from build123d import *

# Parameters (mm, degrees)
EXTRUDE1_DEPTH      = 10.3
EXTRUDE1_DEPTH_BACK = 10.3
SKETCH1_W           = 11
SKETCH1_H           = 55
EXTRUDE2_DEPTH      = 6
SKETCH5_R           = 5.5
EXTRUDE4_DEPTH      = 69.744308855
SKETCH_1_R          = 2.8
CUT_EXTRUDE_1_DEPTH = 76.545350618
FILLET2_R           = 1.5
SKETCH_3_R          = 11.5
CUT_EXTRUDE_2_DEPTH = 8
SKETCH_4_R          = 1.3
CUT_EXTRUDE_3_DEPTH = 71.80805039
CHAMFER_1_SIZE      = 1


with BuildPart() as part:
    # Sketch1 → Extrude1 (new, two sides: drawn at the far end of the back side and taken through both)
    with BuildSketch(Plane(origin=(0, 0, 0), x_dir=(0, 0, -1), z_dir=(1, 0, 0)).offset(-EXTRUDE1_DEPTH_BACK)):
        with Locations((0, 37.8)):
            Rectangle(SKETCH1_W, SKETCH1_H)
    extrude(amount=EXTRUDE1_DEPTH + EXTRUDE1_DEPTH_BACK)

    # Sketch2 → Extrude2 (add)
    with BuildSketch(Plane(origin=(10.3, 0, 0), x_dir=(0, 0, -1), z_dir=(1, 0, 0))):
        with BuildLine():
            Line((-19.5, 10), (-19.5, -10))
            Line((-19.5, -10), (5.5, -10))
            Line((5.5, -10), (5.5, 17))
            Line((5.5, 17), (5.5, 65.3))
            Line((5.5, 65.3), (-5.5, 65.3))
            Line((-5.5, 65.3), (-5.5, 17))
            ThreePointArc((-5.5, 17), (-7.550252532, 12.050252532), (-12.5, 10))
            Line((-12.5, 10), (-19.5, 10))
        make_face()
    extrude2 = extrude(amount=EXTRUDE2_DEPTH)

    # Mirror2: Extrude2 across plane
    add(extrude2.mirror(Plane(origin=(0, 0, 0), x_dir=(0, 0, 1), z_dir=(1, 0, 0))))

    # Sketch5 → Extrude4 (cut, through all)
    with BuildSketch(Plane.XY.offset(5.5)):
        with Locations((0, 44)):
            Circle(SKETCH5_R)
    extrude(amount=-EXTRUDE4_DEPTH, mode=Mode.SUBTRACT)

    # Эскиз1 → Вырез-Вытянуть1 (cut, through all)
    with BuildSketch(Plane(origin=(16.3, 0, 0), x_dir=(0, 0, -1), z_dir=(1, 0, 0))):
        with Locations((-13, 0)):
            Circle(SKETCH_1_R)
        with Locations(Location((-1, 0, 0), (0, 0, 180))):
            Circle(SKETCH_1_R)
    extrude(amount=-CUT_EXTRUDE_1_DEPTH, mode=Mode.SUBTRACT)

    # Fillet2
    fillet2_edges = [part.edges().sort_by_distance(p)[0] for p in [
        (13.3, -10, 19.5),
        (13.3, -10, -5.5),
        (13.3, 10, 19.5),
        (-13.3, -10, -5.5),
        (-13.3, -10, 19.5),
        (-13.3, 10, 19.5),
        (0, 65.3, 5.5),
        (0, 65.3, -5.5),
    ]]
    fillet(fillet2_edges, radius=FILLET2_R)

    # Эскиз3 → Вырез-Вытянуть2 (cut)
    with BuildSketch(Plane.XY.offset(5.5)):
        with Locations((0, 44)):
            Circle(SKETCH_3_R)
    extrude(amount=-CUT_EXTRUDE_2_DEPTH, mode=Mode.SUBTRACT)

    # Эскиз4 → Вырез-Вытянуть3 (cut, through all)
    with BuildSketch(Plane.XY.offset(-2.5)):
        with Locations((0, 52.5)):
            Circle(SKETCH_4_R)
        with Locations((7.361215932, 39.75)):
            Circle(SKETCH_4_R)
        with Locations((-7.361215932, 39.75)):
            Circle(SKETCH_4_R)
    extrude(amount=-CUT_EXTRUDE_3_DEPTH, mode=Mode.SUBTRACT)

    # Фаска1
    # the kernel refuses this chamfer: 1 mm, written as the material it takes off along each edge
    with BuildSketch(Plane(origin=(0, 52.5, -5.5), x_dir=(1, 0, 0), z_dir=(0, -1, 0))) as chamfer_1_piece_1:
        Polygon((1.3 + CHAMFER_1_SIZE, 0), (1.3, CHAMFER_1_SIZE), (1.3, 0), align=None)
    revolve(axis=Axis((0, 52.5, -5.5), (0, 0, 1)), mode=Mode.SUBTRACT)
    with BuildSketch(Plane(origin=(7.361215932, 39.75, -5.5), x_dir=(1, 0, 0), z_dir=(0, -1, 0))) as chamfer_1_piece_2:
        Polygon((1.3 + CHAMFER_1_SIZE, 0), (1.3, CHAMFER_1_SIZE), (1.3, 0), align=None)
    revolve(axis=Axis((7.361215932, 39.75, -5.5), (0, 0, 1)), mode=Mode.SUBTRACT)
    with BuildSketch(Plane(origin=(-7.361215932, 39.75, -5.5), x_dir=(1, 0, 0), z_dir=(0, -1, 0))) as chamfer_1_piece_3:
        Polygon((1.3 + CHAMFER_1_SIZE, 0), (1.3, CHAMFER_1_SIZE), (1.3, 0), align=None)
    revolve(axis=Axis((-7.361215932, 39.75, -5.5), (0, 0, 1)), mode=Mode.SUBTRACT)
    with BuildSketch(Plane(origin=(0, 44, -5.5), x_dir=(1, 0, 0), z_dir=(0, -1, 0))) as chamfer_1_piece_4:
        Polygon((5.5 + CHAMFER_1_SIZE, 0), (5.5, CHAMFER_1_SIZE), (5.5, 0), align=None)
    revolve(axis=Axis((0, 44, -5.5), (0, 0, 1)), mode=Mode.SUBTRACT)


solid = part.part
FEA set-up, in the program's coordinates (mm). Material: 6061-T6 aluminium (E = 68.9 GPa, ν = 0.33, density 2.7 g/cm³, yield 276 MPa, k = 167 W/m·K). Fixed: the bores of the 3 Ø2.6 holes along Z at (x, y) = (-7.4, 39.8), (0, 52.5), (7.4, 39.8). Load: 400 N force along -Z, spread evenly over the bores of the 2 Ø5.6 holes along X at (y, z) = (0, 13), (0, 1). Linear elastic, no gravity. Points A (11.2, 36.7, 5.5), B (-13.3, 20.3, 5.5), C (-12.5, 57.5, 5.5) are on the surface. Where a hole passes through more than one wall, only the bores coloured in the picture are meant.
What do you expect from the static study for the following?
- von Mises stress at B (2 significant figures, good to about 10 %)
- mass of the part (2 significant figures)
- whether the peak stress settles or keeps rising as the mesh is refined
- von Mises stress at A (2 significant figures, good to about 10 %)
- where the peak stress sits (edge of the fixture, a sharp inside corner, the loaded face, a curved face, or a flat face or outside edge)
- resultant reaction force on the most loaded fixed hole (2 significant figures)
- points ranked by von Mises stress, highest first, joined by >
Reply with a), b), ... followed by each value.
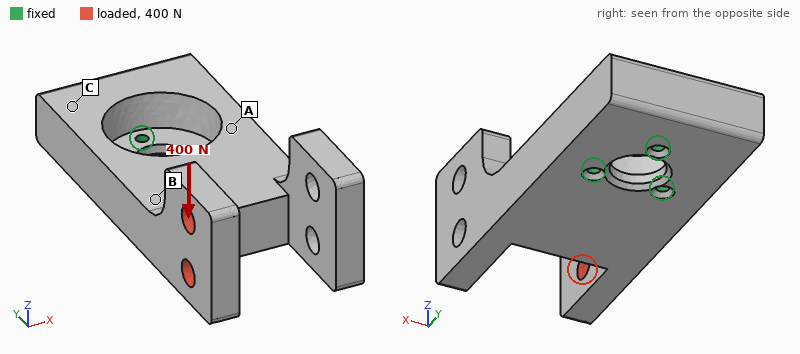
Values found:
a) 25 MPa
b) 58 g
c) keeps rising
d) 45 MPa
e) edge of the fixture
f) 940 N
g) A > B > C
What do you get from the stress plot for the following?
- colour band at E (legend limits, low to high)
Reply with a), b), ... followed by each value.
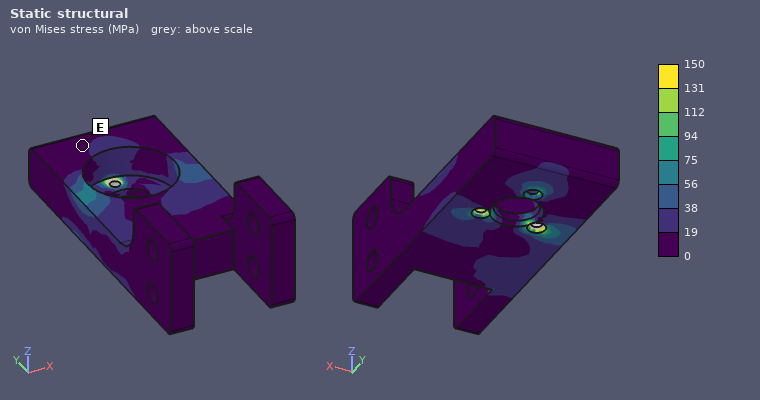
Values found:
a) 0 to 19 MPa
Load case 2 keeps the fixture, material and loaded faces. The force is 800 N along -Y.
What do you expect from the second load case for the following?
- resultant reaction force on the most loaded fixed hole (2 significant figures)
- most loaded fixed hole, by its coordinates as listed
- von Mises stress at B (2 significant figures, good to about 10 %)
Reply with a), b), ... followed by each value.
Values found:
a) 820 N
b) (-7.4, 39.8)
c) 28 MPa
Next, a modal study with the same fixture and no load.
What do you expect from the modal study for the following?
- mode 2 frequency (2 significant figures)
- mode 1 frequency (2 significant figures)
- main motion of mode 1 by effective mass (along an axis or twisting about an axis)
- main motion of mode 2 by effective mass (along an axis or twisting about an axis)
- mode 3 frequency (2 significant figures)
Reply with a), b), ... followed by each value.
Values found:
a) 3500 Hz
b) 1700 Hz
c) along Z
d) along X
e) 4500 Hz
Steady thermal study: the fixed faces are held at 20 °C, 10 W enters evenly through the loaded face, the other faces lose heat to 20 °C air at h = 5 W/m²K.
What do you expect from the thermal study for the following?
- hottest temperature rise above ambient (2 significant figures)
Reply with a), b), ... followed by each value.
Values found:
a) 21 K
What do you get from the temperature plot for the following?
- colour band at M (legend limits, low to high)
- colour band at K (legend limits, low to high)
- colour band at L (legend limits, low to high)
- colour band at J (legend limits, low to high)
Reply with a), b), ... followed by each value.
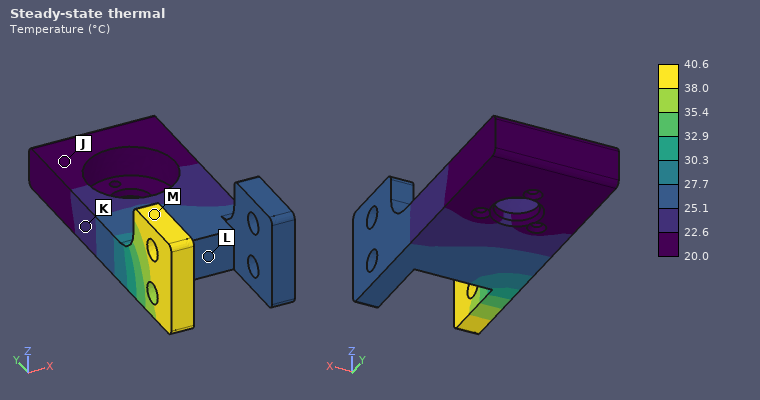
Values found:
a) 38.0 to 40.6 °C
b) 22.6 to 25.1 °C
c) 25.1 to 27.7 °C
d) 20.0 to 22.6 °C
